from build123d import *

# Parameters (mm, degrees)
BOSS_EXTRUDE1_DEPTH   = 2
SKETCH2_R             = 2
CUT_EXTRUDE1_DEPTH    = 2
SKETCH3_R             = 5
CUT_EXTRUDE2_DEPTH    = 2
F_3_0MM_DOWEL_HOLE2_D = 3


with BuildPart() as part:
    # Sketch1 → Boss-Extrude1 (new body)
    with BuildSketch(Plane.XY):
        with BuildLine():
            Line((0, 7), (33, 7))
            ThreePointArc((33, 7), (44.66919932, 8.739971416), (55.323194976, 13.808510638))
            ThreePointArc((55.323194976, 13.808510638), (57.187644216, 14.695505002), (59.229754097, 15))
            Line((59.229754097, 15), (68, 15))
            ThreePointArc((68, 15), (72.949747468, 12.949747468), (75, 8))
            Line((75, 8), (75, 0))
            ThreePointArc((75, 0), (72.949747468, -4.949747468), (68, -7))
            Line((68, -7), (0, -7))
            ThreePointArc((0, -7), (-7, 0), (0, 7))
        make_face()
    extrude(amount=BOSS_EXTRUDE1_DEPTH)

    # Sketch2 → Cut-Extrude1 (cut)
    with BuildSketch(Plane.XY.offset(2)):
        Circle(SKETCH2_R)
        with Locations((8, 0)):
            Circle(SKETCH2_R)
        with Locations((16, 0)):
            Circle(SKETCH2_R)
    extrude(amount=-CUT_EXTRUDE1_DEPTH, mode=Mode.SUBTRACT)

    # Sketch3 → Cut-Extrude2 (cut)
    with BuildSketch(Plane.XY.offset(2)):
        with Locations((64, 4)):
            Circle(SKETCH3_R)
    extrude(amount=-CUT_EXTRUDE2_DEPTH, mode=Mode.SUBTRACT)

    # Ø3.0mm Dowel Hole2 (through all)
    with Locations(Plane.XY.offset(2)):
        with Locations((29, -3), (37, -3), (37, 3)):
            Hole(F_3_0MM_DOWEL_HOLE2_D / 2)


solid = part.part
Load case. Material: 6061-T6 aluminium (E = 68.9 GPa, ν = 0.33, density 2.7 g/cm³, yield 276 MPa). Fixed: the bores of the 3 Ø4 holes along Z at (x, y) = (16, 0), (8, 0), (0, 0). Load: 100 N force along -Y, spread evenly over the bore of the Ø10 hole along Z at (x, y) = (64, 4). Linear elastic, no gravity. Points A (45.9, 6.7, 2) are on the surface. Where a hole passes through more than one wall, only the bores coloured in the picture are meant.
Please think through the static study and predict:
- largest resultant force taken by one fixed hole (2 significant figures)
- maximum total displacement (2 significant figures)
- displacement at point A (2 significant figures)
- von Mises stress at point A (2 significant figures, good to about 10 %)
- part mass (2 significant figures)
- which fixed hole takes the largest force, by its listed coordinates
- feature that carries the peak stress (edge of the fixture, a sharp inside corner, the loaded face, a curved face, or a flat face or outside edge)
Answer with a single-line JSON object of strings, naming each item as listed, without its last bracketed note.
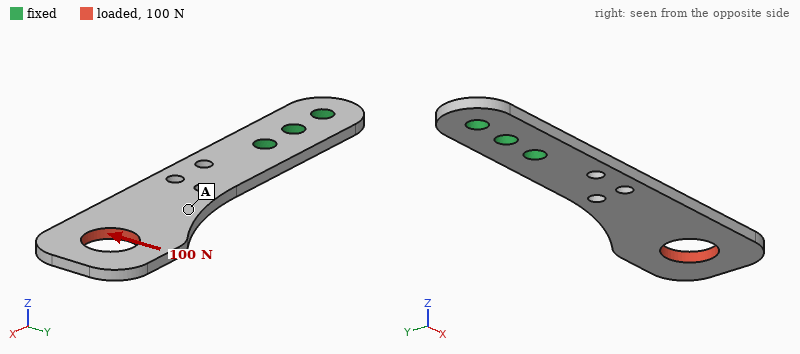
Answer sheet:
{"largest resultant force taken by one fixed hole": "340 N", "maximum total displacement": "0.21 mm", "displacement at point A": "0.086 mm", "von Mises stress at point A": "15 MPa", "part mass": "6.3 g", "which fixed hole takes the largest force, by its listed coordinates": "(16, 0)", "feature that carries the peak stress": "edge of the fixture"}
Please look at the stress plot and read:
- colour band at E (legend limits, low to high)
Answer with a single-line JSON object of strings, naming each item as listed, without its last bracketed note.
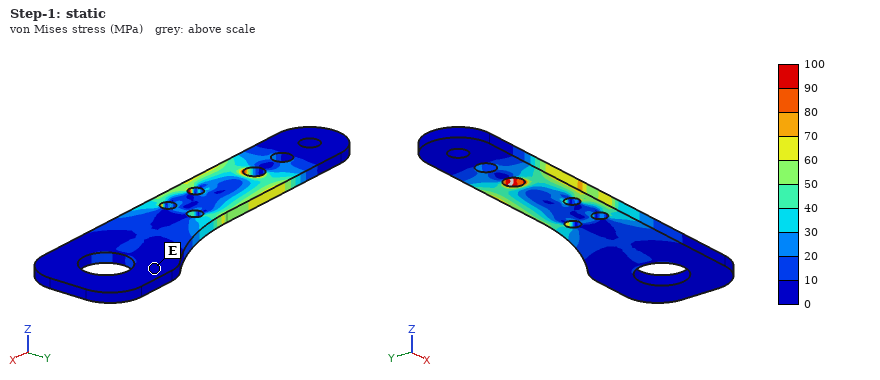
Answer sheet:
{"colour band at E": "0 to 10 MPa"}
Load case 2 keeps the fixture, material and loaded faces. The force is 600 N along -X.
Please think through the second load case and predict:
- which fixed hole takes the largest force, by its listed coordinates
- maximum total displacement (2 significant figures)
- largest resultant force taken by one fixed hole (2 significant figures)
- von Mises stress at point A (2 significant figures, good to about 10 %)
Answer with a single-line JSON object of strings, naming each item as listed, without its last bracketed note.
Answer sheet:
{"which fixed hole takes the largest force, by its listed coordinates": "(16, 0)", "maximum total displacement": "0.13 mm", "largest resultant force taken by one fixed hole": "500 N", "von Mises stress at point A": "33 MPa"}
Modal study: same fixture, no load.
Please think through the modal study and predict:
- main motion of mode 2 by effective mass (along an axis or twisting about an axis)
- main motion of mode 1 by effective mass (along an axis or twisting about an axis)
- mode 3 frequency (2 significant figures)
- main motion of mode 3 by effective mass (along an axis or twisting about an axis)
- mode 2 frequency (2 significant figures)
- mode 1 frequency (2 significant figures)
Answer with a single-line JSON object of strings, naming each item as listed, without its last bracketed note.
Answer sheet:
{"main motion of mode 2 by effective mass": "twisting about X", "main motion of mode 1 by effective mass": "along Z", "mode 3 frequency": "2500 Hz", "main motion of mode 3 by effective mass": "along Y", "mode 2 frequency": "2200 Hz", "mode 1 frequency": "430 Hz"}
